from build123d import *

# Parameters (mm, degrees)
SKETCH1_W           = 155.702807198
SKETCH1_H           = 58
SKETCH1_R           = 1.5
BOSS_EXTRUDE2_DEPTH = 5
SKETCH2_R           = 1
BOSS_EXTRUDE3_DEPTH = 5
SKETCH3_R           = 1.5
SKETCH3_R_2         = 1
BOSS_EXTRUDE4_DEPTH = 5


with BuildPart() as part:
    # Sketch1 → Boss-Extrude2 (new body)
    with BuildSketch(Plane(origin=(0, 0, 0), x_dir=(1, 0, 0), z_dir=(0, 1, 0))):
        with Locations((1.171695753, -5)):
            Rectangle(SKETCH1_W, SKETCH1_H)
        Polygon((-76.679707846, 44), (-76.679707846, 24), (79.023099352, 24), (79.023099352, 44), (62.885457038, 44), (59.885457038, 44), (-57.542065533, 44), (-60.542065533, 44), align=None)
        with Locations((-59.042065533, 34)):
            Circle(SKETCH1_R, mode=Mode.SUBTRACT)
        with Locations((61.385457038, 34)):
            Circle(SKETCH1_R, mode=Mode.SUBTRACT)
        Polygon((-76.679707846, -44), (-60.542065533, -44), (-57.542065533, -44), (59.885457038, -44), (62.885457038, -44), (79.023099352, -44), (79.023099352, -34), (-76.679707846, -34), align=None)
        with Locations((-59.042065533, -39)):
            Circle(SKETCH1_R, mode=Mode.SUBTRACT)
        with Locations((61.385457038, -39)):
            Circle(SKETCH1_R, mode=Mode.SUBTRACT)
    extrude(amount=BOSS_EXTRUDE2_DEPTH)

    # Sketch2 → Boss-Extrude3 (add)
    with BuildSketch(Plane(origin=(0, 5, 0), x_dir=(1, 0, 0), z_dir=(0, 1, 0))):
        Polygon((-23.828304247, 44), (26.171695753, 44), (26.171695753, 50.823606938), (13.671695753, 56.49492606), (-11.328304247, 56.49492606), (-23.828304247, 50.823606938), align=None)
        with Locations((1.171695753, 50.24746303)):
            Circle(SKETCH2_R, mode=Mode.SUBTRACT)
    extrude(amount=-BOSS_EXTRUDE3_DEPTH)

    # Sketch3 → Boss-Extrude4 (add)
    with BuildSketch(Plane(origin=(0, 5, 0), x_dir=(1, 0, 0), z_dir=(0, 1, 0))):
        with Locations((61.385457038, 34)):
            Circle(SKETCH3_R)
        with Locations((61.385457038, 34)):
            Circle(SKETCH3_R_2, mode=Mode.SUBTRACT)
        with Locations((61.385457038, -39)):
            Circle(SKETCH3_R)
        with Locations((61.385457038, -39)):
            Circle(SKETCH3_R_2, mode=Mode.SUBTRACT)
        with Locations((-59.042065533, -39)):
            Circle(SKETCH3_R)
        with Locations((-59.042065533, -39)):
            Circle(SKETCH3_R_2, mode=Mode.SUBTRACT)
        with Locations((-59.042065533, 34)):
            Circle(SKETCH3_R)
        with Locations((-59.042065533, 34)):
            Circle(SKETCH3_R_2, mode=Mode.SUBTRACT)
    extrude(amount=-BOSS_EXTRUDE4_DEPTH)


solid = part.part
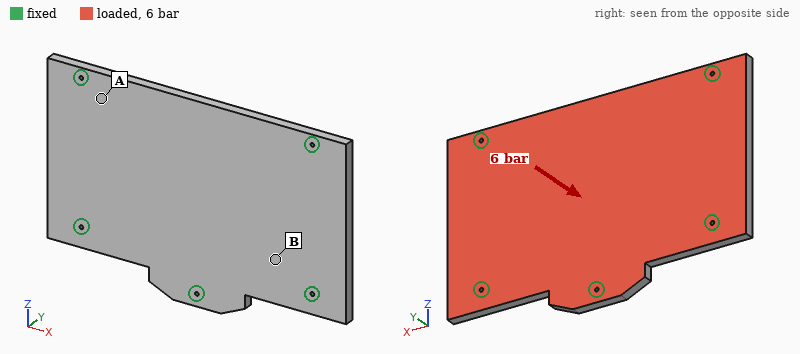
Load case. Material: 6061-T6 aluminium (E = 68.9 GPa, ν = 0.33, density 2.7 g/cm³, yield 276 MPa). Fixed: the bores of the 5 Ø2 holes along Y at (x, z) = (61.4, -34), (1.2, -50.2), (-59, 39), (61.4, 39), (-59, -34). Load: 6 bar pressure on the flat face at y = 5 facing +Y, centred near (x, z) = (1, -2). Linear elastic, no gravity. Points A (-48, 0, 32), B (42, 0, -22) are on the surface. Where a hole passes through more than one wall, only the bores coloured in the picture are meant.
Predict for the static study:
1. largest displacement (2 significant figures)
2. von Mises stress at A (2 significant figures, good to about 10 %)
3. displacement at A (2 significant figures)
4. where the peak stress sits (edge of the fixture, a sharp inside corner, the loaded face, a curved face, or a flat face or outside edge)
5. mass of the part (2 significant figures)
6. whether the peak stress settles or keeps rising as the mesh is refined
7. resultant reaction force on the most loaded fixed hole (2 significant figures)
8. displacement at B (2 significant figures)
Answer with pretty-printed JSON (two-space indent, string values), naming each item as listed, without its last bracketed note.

{
  "largest displacement": "0.71 mm",
  "von Mises stress at A": "78 MPa",
  "displacement at A": "0.15 mm",
  "where the peak stress sits": "edge of the fixture",
  "mass of the part": "190 g",
  "whether the peak stress settles or keeps rising as the mesh is refined": "keeps rising",
  "resultant reaction force on the most loaded fixed hole": "1.9 kN",
  "displacement at B": "0.19 mm"
}
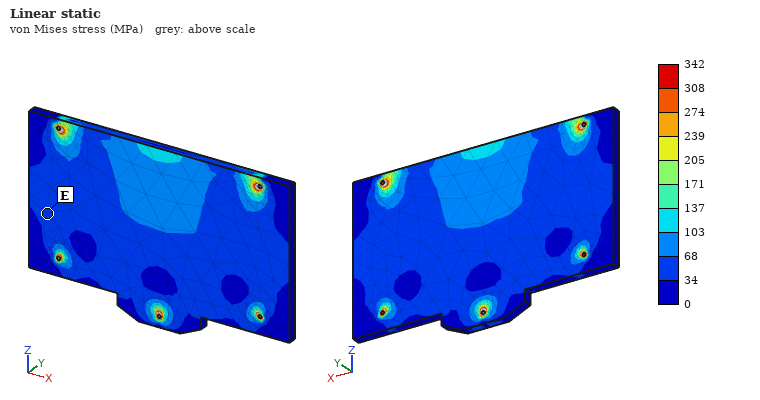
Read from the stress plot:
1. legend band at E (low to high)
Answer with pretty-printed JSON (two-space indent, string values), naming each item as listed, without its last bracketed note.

{
  "legend band at E": "34 to 68 MPa"
}
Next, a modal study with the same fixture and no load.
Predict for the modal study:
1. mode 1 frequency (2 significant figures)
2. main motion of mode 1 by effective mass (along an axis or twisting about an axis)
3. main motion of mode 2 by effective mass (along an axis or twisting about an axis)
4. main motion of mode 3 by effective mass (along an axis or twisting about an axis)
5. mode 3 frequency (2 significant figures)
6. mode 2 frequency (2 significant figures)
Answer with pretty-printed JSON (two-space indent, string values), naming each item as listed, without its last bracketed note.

{
  "mode 1 frequency": "1600 Hz",
  "main motion of mode 1 by effective mass": "along Y",
  "main motion of mode 2 by effective mass": "along Y",
  "main motion of mode 3 by effective mass": "twisting about Z",
  "mode 3 frequency": "3400 Hz",
  "mode 2 frequency": "3200 Hz"
}
